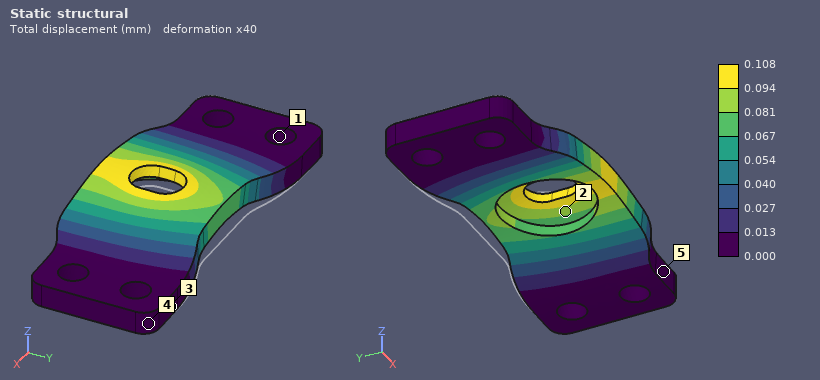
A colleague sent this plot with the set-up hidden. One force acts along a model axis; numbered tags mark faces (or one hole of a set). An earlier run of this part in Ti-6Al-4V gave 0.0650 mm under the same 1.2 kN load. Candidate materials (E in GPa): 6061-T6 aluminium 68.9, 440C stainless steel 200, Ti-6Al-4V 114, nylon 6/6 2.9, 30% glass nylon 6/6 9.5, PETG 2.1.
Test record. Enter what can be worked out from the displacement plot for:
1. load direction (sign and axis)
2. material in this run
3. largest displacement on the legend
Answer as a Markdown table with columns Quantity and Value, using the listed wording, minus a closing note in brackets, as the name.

| Quantity | Value |
|---|---|
| load direction | +Z |
| material in this run | 6061-T6 aluminium |
| largest displacement on the legend | 0.108 mm |
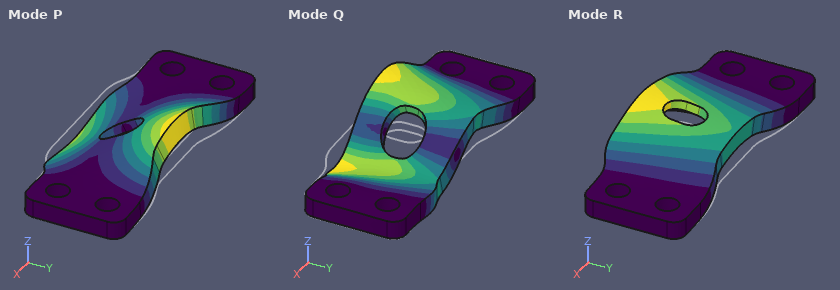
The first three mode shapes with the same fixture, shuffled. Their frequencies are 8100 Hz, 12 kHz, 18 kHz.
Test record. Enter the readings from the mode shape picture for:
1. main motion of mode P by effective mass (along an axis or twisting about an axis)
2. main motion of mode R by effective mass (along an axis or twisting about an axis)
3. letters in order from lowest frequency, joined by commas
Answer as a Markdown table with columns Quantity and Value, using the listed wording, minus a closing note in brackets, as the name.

| Quantity | Value |
|---|---|
| main motion of mode P by effective mass | twisting about X |
| main motion of mode R by effective mass | along Z |
| letters in order from lowest frequency, joined by commas | R, P, Q |
